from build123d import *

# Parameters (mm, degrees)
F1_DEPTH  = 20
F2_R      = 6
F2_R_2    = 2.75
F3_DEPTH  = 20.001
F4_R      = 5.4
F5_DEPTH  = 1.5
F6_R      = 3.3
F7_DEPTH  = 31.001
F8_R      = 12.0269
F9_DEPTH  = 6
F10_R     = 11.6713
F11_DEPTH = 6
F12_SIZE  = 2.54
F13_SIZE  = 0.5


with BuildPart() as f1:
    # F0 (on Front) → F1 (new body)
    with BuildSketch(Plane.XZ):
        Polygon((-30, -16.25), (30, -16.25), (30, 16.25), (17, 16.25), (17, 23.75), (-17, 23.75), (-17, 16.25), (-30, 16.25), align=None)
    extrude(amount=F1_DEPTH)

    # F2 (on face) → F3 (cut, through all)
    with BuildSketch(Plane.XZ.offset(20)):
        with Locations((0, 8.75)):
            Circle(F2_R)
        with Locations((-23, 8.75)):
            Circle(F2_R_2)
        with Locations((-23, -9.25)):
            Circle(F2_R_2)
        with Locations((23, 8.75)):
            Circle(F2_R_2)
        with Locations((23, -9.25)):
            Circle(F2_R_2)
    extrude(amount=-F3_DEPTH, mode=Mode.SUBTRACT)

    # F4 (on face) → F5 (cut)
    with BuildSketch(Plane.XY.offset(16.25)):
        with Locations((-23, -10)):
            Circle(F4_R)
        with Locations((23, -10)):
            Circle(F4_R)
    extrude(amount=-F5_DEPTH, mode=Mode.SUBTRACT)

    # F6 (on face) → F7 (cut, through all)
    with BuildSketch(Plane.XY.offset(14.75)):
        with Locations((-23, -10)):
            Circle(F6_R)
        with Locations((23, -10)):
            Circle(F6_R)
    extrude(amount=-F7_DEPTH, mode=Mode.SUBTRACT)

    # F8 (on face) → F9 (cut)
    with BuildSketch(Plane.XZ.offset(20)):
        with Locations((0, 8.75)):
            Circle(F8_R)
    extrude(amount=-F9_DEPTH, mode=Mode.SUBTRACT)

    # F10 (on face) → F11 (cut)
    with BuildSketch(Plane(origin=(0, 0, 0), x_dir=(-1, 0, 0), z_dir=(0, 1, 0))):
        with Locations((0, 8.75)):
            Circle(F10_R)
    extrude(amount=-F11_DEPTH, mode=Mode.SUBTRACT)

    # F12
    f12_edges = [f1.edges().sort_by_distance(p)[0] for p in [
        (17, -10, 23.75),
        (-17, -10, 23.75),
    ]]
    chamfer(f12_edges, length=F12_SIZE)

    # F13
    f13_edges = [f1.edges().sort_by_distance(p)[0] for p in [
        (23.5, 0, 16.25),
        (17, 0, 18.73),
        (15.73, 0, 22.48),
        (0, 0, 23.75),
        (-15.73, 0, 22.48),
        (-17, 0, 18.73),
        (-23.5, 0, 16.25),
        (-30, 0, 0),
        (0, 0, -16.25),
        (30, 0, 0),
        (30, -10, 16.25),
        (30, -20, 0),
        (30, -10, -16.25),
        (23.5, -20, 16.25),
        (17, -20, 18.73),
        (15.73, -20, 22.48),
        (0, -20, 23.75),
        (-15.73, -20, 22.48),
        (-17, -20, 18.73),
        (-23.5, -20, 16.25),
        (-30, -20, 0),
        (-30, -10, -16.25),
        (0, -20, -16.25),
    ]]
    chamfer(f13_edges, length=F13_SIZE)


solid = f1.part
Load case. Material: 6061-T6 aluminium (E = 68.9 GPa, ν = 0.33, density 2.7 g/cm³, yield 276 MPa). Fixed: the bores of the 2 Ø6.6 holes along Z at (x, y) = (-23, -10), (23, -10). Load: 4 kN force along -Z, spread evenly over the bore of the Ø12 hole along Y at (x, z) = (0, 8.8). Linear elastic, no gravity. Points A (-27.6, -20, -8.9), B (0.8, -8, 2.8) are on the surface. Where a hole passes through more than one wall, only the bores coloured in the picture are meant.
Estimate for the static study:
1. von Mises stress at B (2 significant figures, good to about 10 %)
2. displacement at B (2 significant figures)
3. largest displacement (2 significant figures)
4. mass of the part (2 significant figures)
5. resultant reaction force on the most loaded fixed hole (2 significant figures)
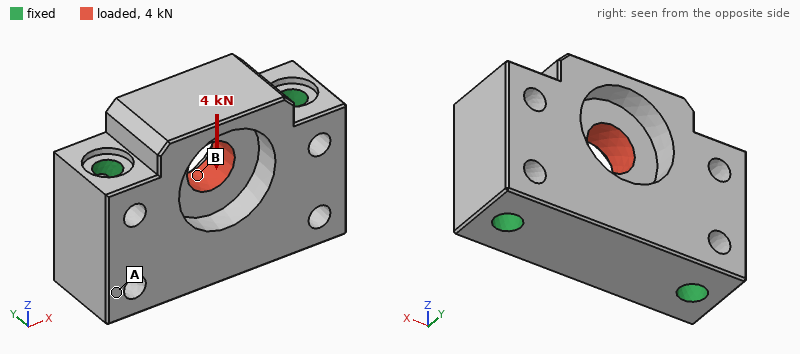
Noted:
12 MPa
3.7 µm
5.8 µm
92 g
2.1 kN
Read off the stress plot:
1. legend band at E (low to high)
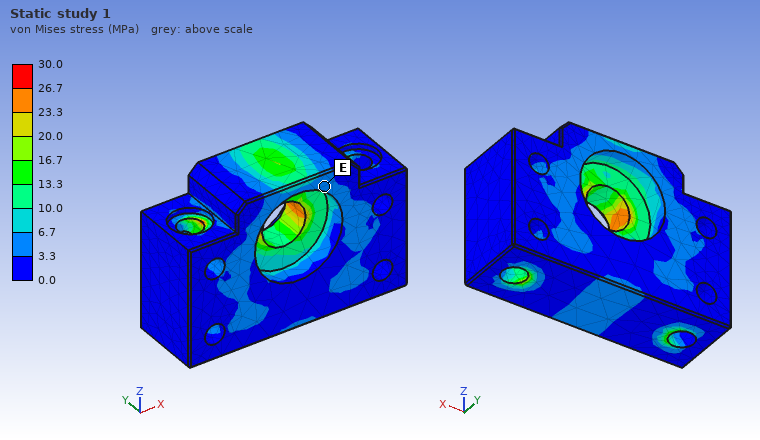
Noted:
3.3 to 6.7 MPa
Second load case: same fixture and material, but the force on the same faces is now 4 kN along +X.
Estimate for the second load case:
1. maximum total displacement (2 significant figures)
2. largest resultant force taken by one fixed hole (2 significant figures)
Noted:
3.7 µm
2.0 kN
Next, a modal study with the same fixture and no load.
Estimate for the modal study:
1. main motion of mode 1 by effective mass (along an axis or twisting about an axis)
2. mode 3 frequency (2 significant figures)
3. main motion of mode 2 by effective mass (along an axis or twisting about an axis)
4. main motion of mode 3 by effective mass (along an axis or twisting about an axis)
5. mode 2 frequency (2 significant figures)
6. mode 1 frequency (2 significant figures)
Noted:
along Y
31 kHz
along Y
along Z
25 kHz
19 kHz
